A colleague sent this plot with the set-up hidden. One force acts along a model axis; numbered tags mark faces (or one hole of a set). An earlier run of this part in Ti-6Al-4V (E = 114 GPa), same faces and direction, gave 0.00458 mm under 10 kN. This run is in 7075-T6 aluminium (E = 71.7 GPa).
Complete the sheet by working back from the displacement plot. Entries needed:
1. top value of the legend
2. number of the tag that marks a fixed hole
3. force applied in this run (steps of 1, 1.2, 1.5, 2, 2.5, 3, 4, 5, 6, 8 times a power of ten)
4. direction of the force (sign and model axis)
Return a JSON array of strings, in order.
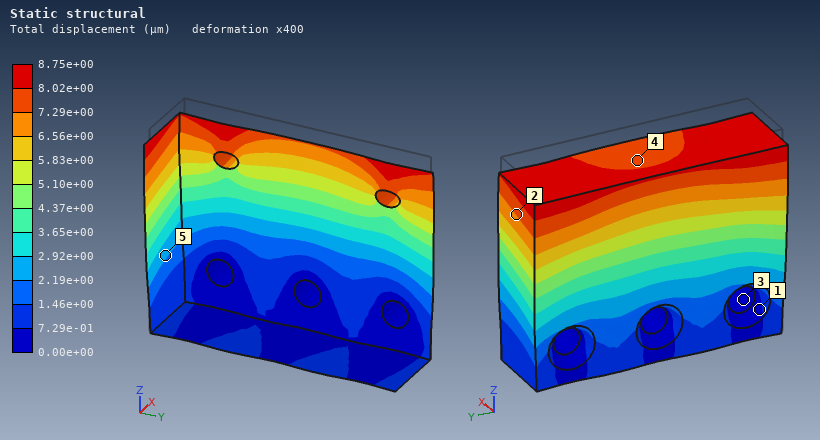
["8.75e+00 µm", "3", "12 kN", "-Z"]
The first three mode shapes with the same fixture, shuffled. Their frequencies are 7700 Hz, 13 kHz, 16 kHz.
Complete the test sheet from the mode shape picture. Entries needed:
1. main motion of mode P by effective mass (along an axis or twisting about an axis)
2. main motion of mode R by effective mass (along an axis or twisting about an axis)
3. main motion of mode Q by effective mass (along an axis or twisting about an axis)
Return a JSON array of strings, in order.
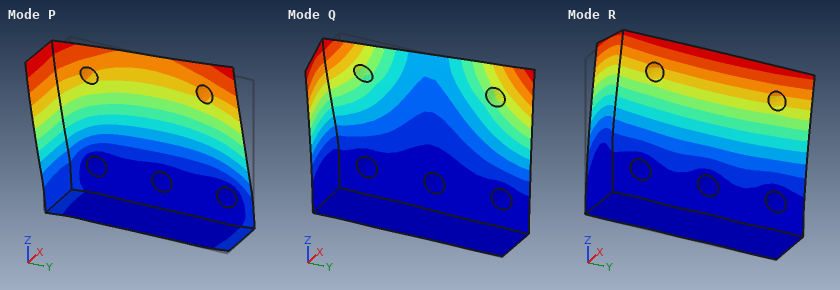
["along Y", "along X", "twisting about Z"]
